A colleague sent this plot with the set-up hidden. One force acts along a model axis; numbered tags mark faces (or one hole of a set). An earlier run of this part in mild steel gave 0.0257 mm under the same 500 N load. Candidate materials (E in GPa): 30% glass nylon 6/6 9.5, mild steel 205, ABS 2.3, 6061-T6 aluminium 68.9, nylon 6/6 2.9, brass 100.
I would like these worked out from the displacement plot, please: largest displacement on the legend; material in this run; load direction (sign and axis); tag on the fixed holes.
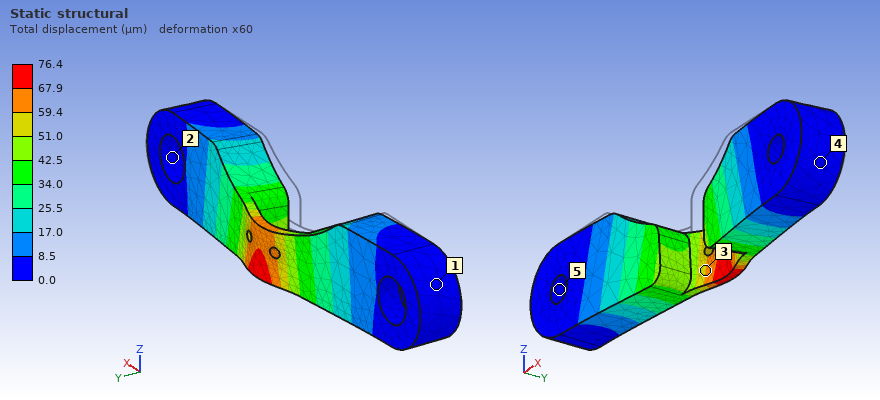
76.4 µm
6061-T6 aluminium
+Y
5
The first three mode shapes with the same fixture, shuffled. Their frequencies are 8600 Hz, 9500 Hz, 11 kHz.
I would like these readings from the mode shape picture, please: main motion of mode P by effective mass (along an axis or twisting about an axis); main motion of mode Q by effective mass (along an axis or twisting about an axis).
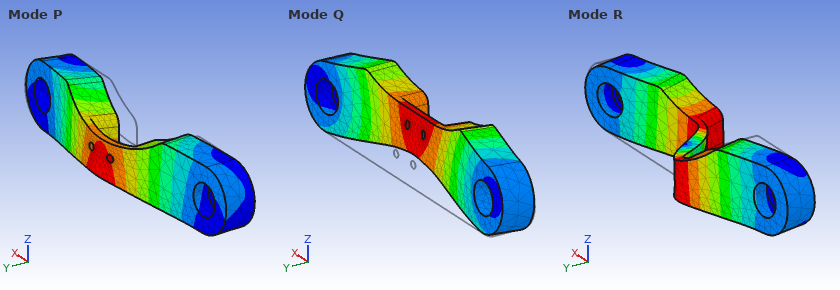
along Y
along Z
